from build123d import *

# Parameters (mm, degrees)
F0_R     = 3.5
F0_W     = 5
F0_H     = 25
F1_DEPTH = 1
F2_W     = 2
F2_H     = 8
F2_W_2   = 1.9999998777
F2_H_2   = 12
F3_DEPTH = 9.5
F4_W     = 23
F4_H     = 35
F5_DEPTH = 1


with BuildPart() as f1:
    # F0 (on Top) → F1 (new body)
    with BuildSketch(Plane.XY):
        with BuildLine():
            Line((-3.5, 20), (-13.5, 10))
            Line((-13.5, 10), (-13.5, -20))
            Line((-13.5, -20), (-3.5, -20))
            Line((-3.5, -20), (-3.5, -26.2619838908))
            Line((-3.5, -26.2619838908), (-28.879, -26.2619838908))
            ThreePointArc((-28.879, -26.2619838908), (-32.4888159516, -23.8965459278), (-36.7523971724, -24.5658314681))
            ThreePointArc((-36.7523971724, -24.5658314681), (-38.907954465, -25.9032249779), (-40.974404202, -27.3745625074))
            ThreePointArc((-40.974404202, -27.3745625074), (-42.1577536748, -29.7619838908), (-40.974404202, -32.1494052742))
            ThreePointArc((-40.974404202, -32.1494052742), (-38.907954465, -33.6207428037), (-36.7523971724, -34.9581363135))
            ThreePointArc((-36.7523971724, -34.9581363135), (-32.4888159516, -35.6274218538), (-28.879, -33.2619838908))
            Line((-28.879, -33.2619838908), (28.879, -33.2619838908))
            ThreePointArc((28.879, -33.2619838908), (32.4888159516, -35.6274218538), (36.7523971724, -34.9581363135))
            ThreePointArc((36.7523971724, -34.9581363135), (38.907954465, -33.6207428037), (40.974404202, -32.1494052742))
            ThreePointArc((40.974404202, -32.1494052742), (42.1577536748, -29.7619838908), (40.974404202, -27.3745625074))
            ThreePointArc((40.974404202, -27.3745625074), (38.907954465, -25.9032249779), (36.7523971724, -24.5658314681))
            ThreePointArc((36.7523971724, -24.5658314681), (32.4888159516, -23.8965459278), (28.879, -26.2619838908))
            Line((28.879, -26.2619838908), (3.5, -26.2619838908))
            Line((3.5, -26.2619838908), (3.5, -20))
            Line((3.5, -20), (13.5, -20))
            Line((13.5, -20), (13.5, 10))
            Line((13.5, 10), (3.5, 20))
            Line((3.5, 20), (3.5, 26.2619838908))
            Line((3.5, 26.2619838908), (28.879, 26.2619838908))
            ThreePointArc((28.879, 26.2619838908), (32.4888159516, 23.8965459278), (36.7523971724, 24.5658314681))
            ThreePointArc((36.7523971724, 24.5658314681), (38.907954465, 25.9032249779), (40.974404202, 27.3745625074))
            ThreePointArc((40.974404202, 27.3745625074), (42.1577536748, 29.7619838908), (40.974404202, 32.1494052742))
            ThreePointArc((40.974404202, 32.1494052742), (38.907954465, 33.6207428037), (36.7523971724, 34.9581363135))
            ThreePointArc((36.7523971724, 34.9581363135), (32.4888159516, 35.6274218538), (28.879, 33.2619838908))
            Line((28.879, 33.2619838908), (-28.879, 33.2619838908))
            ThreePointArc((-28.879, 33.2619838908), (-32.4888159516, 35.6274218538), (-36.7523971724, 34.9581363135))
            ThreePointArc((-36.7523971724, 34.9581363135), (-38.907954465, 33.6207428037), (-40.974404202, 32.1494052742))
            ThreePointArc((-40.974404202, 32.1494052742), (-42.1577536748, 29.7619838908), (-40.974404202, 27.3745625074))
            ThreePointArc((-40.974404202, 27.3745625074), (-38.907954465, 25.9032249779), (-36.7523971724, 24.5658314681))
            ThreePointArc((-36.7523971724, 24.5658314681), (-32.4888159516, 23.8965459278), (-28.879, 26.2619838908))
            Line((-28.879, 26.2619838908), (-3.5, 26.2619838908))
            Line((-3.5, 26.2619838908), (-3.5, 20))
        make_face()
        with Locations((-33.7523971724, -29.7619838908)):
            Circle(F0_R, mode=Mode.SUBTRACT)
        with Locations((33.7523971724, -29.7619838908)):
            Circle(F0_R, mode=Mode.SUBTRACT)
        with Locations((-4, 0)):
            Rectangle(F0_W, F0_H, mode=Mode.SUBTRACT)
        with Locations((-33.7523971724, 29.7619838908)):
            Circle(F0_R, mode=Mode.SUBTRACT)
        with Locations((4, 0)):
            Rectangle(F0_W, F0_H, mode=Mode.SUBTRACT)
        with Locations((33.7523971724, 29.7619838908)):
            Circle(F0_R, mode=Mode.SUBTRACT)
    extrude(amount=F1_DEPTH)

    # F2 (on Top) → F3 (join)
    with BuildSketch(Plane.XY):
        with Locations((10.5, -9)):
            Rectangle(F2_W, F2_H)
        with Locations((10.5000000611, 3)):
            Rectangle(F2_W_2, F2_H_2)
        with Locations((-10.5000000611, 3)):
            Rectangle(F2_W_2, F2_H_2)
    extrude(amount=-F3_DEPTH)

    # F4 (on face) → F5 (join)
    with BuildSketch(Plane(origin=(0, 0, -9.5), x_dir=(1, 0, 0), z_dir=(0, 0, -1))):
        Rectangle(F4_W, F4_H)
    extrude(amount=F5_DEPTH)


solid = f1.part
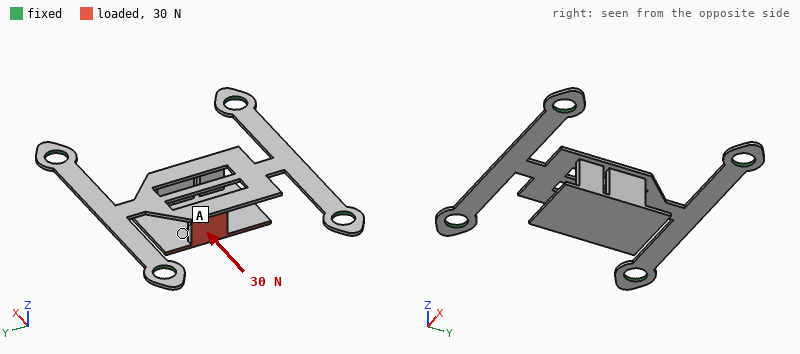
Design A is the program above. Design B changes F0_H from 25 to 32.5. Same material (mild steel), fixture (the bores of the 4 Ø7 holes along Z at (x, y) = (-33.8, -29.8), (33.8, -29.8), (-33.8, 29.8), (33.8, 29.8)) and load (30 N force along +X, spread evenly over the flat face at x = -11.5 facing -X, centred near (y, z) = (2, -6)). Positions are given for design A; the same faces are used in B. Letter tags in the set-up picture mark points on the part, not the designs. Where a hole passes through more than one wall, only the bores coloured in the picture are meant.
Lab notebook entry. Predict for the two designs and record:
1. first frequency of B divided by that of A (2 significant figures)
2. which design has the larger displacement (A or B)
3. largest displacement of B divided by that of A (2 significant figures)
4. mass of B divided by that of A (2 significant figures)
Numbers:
0.98
B
1.1
0.98
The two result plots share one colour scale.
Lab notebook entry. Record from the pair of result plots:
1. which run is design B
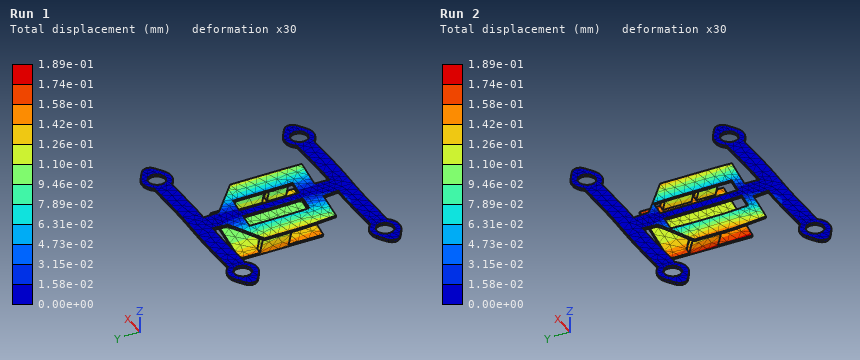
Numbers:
Run 2
